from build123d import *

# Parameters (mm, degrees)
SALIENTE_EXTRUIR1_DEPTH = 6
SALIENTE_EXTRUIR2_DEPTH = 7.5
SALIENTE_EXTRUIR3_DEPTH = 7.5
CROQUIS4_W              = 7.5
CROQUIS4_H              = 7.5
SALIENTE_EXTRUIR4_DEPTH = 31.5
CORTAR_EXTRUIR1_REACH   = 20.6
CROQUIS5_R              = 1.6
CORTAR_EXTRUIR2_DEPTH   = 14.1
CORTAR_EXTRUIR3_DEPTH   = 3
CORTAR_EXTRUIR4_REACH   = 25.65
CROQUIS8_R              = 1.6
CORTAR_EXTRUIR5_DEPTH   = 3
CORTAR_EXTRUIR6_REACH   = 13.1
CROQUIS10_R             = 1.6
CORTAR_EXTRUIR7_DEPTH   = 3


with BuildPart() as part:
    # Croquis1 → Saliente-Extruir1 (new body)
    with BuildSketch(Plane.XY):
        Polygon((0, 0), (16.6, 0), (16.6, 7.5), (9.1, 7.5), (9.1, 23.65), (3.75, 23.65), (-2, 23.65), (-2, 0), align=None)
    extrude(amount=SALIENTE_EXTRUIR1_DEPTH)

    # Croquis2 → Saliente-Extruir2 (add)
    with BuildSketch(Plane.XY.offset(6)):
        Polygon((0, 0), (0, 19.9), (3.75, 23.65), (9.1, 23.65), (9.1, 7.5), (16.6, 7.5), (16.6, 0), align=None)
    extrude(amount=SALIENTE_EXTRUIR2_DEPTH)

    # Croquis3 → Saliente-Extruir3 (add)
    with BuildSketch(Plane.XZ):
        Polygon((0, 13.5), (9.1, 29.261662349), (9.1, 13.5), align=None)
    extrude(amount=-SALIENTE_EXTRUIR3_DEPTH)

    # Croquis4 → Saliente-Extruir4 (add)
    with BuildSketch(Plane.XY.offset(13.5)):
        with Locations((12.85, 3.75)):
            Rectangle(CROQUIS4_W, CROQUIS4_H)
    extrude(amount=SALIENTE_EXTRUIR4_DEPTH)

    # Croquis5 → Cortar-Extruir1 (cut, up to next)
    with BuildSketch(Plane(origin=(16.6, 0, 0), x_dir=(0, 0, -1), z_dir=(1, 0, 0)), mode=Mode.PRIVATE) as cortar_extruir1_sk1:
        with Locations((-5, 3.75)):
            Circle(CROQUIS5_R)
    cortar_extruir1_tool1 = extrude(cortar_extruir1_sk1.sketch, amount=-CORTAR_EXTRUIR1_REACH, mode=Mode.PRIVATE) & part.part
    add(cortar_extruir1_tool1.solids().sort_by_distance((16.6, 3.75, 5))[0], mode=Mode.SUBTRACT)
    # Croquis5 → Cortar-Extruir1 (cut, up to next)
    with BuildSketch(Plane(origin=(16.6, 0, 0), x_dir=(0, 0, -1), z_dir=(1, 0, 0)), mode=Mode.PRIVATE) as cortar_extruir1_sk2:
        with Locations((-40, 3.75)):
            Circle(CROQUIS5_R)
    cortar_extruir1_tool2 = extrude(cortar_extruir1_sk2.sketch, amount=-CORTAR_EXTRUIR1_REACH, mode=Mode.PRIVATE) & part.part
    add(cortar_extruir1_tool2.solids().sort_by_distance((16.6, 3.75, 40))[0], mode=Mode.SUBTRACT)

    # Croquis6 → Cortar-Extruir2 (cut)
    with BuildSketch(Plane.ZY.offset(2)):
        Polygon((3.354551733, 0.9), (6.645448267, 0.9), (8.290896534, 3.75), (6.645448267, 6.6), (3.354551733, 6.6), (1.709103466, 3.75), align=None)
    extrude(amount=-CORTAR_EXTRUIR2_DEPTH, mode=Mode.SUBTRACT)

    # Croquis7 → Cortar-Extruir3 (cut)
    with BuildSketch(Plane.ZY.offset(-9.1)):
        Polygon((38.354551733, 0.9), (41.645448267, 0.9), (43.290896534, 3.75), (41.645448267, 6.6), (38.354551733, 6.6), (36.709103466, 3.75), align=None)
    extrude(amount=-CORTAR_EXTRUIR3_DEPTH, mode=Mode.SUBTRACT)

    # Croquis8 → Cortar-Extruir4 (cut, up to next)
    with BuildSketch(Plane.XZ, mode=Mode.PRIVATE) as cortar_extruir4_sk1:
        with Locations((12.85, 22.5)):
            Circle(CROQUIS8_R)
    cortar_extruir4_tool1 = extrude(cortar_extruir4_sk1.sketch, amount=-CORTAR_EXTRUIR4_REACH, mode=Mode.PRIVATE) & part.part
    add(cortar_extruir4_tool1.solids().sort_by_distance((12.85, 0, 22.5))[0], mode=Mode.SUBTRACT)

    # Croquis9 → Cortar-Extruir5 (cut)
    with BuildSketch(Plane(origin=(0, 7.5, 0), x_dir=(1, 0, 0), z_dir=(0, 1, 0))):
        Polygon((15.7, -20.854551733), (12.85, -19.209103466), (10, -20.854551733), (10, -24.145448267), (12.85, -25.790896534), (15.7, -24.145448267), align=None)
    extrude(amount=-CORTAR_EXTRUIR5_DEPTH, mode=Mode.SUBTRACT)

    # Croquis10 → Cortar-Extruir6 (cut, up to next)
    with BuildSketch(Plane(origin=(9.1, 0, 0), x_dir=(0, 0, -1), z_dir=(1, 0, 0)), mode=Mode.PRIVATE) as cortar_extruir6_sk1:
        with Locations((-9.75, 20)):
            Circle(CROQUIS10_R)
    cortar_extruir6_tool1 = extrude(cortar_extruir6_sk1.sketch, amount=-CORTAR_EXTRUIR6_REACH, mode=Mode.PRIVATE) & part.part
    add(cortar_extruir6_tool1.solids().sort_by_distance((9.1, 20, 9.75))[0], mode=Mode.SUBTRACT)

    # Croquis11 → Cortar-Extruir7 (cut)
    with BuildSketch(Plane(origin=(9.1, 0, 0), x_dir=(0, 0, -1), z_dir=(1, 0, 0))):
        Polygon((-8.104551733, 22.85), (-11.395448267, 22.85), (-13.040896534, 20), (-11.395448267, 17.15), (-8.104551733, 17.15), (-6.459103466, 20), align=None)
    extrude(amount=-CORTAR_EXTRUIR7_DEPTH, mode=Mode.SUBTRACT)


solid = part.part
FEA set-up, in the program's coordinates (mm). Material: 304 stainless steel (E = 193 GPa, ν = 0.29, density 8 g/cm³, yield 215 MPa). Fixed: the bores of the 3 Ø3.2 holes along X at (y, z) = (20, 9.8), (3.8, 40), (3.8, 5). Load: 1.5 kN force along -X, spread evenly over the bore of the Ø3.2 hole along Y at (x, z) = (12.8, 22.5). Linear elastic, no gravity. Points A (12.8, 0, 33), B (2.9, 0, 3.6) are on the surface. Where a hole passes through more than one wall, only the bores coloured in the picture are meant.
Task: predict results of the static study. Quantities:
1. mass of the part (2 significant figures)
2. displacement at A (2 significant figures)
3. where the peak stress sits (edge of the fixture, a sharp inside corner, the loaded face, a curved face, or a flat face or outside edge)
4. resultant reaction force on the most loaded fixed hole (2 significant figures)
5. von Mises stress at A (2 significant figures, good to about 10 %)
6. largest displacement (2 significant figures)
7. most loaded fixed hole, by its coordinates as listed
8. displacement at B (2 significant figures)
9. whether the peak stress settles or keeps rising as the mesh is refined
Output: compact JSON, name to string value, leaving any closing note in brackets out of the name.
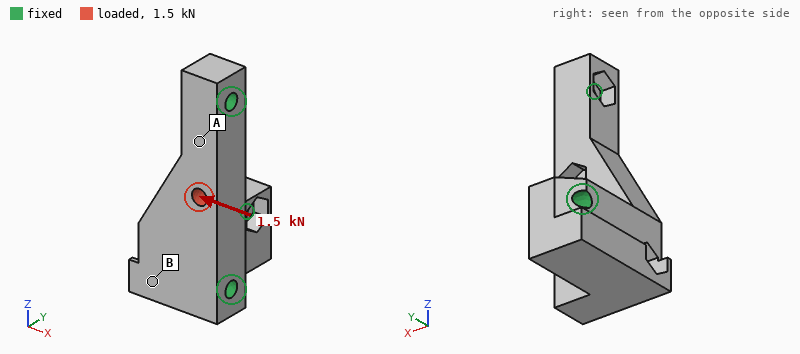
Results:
{"mass of the part": "43 g", "displacement at A": "4.2 µm", "where the peak stress sits": "edge of the fixture", "resultant reaction force on the most loaded fixed hole": "980 N", "von Mises stress at A": "41 MPa", "largest displacement": "9.0 µm", "most loaded fixed hole, by its coordinates as listed": "(3.8, 5)", "displacement at B": "2.9 µm", "whether the peak stress settles or keeps rising as the mesh is refined": "keeps rising"}
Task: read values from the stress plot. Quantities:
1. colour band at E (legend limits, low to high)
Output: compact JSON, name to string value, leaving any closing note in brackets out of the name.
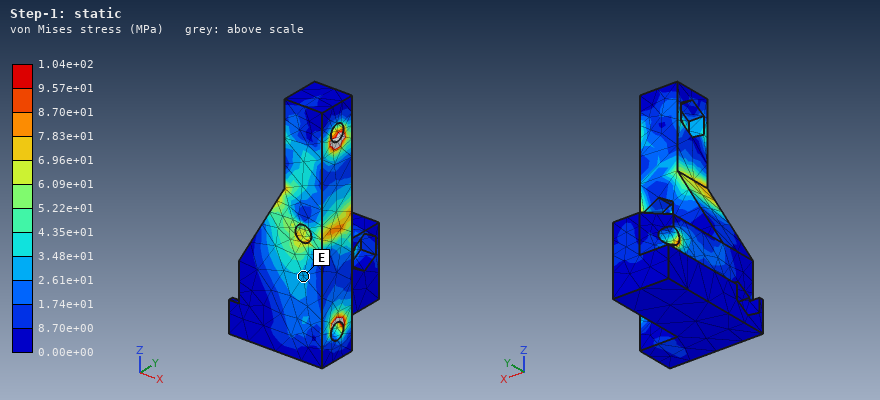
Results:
{"colour band at E": "2.61e+01 to 3.48e+01 MPa"}
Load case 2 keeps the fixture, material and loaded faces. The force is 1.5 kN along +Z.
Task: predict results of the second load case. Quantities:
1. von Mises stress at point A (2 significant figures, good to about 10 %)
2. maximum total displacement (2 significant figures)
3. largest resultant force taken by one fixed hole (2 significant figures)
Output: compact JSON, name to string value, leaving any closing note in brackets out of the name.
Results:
{"von Mises stress at point A": "18 MPa", "maximum total displacement": "1.8 µm", "largest resultant force taken by one fixed hole": "740 N"}
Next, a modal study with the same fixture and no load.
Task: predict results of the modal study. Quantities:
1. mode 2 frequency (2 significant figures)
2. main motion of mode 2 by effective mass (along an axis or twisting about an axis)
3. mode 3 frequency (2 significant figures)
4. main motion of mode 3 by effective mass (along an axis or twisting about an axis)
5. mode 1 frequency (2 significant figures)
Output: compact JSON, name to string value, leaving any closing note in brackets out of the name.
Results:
{"mode 2 frequency": "24 kHz", "main motion of mode 2 by effective mass": "along Y", "mode 3 frequency": "32 kHz", "main motion of mode 3 by effective mass": "along X", "mode 1 frequency": "21 kHz"}
